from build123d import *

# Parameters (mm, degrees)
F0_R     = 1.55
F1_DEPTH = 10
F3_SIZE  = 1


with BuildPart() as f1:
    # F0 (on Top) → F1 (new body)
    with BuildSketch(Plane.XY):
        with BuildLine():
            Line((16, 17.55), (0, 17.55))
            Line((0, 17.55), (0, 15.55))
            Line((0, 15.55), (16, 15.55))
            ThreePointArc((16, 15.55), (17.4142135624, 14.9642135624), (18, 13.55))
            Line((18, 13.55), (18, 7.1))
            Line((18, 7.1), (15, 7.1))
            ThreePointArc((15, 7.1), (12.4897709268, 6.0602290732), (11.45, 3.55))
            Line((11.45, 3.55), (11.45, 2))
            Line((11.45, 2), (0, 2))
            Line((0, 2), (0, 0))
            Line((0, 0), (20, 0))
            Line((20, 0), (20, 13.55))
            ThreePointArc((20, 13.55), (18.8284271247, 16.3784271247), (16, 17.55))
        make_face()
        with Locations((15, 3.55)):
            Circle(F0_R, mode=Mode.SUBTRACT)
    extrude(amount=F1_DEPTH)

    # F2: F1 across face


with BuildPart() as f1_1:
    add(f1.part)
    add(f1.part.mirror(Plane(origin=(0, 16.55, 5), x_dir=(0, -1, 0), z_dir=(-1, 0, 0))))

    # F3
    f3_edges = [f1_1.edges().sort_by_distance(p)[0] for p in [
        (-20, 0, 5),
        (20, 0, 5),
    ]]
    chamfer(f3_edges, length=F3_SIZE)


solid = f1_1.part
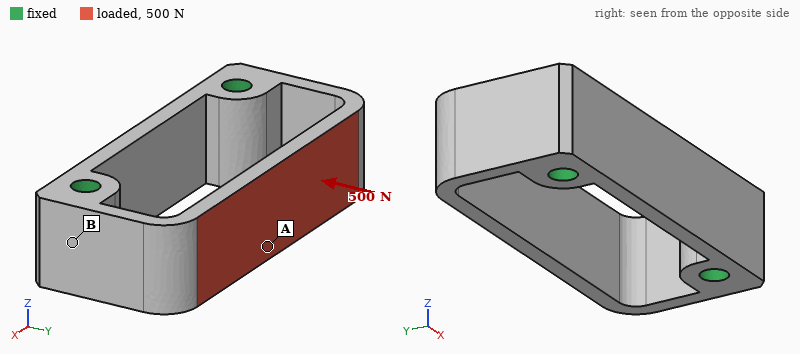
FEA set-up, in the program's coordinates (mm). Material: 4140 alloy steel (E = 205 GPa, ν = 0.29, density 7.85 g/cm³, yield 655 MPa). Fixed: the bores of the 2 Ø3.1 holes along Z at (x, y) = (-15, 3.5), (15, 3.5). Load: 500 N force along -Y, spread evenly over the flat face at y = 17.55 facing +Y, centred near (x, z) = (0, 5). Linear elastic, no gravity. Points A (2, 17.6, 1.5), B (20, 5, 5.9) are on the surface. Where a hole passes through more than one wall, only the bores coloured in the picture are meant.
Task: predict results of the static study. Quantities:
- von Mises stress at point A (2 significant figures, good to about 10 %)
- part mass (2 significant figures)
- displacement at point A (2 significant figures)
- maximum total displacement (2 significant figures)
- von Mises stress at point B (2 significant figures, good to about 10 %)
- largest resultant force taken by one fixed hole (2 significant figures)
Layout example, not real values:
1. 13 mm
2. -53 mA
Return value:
1. 160 MPa
2. 20 g
3. 77 µm
4. 80 µm
5. 39 MPa
6. 360 N
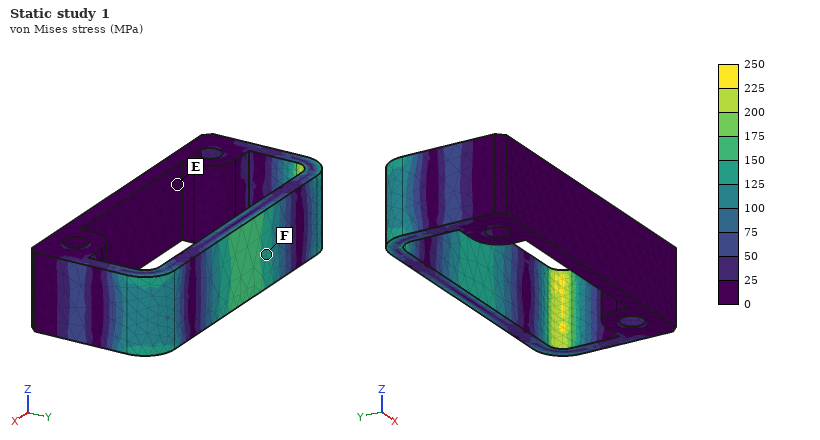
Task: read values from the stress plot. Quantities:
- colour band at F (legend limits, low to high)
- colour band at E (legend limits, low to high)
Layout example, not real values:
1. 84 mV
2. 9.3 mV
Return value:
1. 125 to 150 MPa
2. 0 to 25 MPa
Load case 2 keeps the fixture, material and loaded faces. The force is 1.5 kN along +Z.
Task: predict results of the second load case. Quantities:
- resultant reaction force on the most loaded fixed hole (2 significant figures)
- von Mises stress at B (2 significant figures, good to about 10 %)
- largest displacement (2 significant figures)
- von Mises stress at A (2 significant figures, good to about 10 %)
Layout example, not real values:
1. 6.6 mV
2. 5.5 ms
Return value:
1. 750 N
2. 80 MPa
3. 75 µm
4. 140 MPa
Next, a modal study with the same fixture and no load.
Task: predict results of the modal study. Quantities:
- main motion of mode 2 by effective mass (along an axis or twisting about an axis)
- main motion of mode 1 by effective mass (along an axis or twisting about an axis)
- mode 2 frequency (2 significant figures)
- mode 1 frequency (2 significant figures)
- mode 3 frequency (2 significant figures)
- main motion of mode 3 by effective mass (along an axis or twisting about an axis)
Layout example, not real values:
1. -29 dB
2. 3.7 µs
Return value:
1. along X
2. along Y
3. 7000 Hz
4. 6400 Hz
5. 11 kHz
6. along Z
